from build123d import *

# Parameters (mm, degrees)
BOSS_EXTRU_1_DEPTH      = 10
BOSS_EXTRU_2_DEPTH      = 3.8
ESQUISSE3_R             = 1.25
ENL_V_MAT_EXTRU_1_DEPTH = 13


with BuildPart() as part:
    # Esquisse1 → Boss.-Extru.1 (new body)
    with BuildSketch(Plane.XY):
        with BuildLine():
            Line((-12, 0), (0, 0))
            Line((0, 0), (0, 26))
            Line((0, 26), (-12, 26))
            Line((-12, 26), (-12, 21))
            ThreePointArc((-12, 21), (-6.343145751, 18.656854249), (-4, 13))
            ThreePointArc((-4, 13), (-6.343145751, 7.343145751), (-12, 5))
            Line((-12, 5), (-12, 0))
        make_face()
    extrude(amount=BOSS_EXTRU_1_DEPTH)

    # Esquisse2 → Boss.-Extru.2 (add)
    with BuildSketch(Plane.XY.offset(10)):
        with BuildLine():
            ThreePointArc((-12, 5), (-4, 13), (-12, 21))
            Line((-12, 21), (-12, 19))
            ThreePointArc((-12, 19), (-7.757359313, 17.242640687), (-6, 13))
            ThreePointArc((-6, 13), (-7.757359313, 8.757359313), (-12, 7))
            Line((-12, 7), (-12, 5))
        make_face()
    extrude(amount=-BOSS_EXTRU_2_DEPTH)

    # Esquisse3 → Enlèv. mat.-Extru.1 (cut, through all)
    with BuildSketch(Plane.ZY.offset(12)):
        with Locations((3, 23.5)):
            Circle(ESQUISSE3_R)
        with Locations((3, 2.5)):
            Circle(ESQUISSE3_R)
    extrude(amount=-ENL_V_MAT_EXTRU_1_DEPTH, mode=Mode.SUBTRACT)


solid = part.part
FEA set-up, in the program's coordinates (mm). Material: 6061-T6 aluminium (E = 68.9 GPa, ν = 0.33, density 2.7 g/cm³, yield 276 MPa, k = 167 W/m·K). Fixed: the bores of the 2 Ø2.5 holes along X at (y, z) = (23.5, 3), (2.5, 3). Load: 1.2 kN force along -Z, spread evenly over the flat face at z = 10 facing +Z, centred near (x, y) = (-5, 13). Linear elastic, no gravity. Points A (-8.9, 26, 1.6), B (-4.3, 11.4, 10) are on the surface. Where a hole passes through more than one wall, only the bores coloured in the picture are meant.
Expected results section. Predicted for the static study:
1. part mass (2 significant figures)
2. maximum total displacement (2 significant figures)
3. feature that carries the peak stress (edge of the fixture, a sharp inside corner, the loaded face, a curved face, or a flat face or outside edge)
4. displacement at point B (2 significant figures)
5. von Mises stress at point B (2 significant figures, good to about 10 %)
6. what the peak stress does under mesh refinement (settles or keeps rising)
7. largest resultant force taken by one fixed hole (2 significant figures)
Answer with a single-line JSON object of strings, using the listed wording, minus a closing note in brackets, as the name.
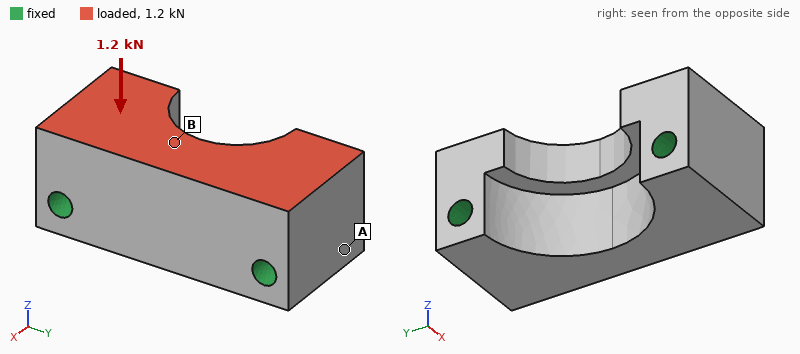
{"part mass": "5.8 g", "maximum total displacement": "2.4 µm", "feature that carries the peak stress": "edge of the fixture", "displacement at point B": "2.2 µm", "von Mises stress at point B": "11 MPa", "what the peak stress does under mesh refinement": "keeps rising", "largest resultant force taken by one fixed hole": "620 N"}
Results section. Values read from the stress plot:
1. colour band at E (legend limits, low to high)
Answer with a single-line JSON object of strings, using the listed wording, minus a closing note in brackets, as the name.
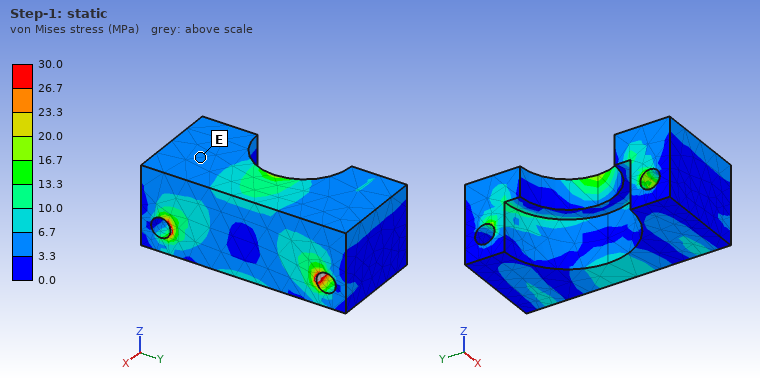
{"colour band at E": "3.3 to 6.7 MPa"}
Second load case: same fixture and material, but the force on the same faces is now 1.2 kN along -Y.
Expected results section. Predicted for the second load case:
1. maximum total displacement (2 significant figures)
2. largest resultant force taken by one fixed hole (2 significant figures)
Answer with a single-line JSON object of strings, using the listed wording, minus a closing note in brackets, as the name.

{"maximum total displacement": "4.8 µm", "largest resultant force taken by one fixed hole": "670 N"}
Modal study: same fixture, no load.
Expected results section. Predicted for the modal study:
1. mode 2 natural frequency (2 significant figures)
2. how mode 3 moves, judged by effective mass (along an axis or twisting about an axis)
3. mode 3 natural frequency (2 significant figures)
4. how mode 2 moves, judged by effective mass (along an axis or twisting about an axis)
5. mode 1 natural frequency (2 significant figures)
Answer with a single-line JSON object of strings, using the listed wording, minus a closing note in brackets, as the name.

{"mode 2 natural frequency": "61 kHz", "how mode 3 moves, judged by effective mass": "along Y", "mode 3 natural frequency": "70 kHz", "how mode 2 moves, judged by effective mass": "along X", "mode 1 natural frequency": "51 kHz"}
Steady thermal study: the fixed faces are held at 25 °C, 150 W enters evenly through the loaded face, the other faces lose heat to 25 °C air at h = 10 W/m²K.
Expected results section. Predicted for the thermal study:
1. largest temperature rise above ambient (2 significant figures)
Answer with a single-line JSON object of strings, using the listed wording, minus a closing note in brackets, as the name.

{"largest temperature rise above ambient": "40 K"}
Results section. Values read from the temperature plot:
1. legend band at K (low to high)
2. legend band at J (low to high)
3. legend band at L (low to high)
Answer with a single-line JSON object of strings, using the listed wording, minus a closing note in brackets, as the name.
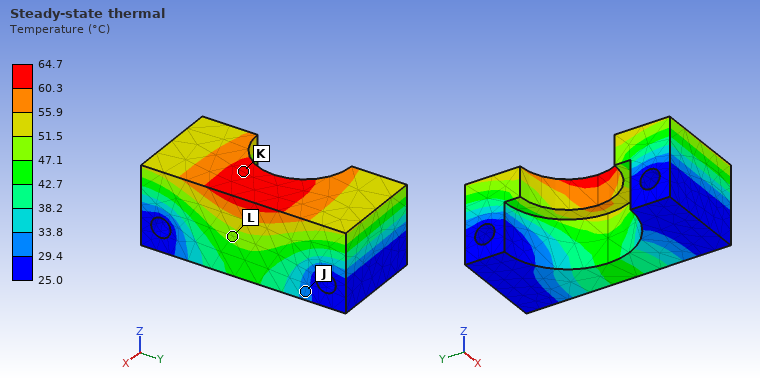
{"legend band at K": "60.3 to 64.7 °C", "legend band at J": "29.4 to 33.8 °C", "legend band at L": "47.1 to 51.5 °C"}
